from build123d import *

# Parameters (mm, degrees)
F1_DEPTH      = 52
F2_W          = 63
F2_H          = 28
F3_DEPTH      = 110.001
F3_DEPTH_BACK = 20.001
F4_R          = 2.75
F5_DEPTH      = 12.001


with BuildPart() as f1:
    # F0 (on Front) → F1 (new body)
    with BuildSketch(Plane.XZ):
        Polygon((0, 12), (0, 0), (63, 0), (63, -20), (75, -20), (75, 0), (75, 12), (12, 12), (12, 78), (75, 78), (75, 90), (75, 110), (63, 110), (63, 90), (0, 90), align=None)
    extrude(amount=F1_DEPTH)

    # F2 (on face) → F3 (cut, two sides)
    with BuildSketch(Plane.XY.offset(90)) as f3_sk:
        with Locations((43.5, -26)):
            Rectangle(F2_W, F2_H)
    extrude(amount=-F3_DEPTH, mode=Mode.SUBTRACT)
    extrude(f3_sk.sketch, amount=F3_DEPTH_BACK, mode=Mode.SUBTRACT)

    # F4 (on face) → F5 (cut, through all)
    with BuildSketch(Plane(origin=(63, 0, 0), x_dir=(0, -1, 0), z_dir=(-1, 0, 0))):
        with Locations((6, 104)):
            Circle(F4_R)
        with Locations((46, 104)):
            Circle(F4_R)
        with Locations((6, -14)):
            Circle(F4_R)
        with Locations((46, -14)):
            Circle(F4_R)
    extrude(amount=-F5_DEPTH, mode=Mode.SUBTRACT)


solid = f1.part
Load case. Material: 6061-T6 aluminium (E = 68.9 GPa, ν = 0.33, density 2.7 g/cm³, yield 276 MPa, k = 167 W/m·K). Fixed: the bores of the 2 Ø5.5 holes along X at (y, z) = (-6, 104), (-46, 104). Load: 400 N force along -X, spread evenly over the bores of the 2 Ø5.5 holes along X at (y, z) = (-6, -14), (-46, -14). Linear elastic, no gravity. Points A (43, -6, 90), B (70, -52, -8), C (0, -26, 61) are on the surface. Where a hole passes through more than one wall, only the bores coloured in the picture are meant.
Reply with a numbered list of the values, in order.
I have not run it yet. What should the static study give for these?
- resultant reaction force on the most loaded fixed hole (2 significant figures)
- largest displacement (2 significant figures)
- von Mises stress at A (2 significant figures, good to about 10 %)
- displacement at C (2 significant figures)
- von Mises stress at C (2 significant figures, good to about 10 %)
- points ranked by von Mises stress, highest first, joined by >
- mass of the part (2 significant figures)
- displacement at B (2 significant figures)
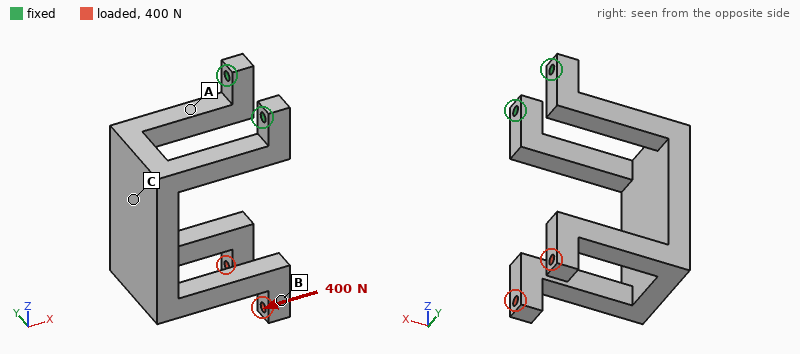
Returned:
1. 200 N
2. 1.8 mm
3. 67 MPa
4. 0.69 mm
5. 23 MPa
6. A > C > B
7. 280 g
8. 1.6 mm
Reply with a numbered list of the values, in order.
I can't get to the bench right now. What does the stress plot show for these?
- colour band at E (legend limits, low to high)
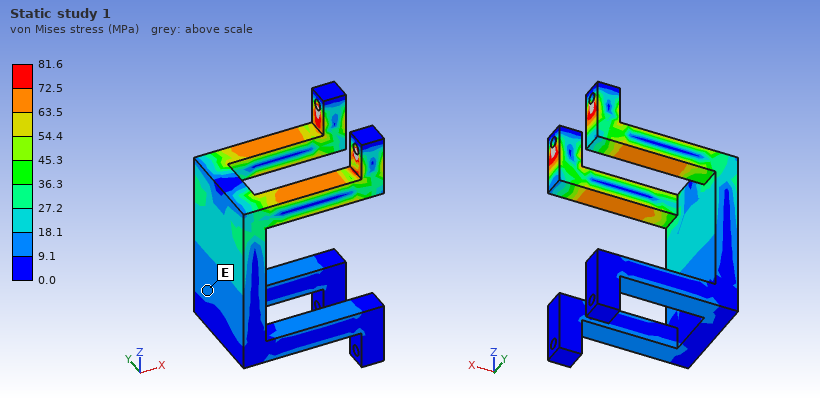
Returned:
1. 9.1 to 18.1 MPa
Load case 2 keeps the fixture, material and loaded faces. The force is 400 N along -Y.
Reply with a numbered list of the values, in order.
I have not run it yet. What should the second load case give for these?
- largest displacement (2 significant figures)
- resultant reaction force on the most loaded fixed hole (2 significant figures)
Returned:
1. 1.6 mm
2. 540 N
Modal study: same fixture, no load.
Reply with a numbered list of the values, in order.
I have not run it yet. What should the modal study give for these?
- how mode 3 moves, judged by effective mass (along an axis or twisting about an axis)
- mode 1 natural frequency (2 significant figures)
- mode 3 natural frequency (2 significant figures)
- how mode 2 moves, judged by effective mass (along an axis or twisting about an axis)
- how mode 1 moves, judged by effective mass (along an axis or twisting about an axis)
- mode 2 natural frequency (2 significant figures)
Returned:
1. along Z
2. 260 Hz
3. 700 Hz
4. along Y
5. along X
6. 340 Hz
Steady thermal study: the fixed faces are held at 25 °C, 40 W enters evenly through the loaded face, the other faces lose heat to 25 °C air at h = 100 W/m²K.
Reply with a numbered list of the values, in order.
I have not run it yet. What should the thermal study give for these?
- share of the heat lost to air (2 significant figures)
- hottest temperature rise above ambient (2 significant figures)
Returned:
1. 92 %
2. 50 K
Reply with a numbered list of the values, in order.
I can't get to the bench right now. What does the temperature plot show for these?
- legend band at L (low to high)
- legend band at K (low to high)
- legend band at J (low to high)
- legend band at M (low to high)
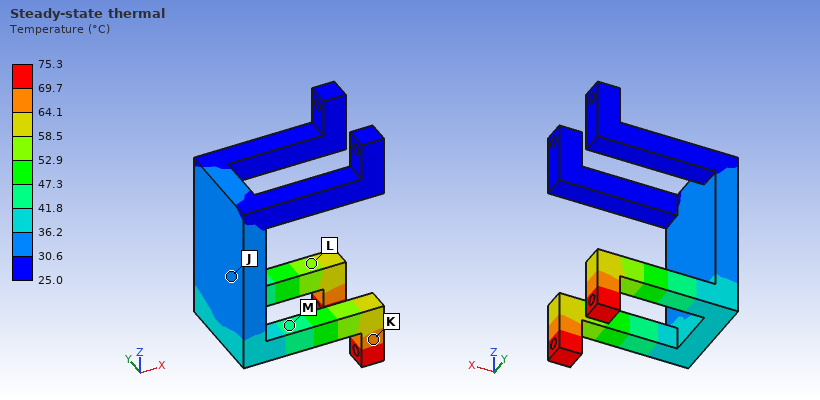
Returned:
1. 52.9 to 58.5 °C
2. 64.1 to 69.7 °C
3. 30.6 to 36.2 °C
4. 41.8 to 47.3 °C
